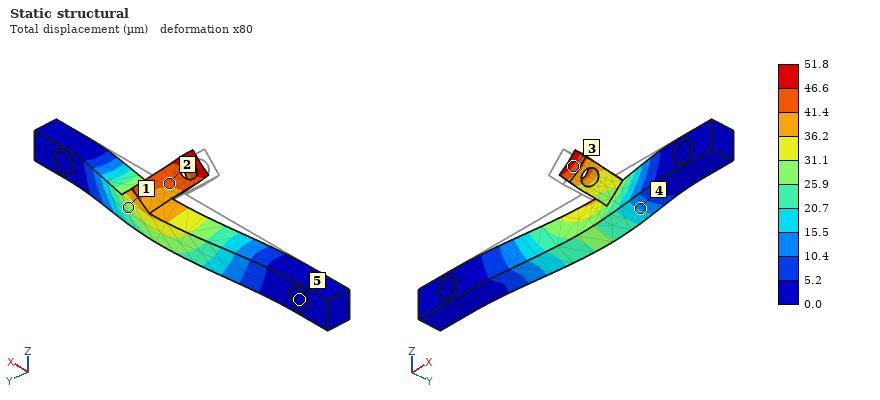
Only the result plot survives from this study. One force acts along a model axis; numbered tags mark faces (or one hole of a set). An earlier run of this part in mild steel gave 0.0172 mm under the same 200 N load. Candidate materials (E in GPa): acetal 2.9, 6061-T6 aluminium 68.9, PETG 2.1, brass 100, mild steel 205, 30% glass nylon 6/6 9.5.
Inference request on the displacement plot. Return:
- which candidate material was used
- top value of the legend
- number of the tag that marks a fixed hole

6061-T6 aluminium
51.8 µm
5
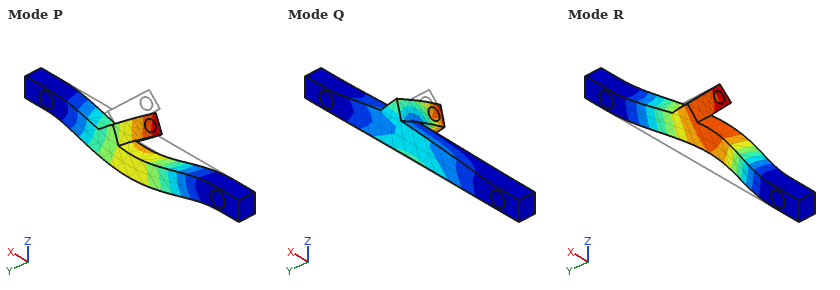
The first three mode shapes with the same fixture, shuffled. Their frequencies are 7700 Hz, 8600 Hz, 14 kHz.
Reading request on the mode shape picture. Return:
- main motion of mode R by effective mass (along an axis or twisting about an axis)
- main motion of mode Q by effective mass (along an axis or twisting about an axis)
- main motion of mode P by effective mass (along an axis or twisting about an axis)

along Y
twisting about X
along Z
